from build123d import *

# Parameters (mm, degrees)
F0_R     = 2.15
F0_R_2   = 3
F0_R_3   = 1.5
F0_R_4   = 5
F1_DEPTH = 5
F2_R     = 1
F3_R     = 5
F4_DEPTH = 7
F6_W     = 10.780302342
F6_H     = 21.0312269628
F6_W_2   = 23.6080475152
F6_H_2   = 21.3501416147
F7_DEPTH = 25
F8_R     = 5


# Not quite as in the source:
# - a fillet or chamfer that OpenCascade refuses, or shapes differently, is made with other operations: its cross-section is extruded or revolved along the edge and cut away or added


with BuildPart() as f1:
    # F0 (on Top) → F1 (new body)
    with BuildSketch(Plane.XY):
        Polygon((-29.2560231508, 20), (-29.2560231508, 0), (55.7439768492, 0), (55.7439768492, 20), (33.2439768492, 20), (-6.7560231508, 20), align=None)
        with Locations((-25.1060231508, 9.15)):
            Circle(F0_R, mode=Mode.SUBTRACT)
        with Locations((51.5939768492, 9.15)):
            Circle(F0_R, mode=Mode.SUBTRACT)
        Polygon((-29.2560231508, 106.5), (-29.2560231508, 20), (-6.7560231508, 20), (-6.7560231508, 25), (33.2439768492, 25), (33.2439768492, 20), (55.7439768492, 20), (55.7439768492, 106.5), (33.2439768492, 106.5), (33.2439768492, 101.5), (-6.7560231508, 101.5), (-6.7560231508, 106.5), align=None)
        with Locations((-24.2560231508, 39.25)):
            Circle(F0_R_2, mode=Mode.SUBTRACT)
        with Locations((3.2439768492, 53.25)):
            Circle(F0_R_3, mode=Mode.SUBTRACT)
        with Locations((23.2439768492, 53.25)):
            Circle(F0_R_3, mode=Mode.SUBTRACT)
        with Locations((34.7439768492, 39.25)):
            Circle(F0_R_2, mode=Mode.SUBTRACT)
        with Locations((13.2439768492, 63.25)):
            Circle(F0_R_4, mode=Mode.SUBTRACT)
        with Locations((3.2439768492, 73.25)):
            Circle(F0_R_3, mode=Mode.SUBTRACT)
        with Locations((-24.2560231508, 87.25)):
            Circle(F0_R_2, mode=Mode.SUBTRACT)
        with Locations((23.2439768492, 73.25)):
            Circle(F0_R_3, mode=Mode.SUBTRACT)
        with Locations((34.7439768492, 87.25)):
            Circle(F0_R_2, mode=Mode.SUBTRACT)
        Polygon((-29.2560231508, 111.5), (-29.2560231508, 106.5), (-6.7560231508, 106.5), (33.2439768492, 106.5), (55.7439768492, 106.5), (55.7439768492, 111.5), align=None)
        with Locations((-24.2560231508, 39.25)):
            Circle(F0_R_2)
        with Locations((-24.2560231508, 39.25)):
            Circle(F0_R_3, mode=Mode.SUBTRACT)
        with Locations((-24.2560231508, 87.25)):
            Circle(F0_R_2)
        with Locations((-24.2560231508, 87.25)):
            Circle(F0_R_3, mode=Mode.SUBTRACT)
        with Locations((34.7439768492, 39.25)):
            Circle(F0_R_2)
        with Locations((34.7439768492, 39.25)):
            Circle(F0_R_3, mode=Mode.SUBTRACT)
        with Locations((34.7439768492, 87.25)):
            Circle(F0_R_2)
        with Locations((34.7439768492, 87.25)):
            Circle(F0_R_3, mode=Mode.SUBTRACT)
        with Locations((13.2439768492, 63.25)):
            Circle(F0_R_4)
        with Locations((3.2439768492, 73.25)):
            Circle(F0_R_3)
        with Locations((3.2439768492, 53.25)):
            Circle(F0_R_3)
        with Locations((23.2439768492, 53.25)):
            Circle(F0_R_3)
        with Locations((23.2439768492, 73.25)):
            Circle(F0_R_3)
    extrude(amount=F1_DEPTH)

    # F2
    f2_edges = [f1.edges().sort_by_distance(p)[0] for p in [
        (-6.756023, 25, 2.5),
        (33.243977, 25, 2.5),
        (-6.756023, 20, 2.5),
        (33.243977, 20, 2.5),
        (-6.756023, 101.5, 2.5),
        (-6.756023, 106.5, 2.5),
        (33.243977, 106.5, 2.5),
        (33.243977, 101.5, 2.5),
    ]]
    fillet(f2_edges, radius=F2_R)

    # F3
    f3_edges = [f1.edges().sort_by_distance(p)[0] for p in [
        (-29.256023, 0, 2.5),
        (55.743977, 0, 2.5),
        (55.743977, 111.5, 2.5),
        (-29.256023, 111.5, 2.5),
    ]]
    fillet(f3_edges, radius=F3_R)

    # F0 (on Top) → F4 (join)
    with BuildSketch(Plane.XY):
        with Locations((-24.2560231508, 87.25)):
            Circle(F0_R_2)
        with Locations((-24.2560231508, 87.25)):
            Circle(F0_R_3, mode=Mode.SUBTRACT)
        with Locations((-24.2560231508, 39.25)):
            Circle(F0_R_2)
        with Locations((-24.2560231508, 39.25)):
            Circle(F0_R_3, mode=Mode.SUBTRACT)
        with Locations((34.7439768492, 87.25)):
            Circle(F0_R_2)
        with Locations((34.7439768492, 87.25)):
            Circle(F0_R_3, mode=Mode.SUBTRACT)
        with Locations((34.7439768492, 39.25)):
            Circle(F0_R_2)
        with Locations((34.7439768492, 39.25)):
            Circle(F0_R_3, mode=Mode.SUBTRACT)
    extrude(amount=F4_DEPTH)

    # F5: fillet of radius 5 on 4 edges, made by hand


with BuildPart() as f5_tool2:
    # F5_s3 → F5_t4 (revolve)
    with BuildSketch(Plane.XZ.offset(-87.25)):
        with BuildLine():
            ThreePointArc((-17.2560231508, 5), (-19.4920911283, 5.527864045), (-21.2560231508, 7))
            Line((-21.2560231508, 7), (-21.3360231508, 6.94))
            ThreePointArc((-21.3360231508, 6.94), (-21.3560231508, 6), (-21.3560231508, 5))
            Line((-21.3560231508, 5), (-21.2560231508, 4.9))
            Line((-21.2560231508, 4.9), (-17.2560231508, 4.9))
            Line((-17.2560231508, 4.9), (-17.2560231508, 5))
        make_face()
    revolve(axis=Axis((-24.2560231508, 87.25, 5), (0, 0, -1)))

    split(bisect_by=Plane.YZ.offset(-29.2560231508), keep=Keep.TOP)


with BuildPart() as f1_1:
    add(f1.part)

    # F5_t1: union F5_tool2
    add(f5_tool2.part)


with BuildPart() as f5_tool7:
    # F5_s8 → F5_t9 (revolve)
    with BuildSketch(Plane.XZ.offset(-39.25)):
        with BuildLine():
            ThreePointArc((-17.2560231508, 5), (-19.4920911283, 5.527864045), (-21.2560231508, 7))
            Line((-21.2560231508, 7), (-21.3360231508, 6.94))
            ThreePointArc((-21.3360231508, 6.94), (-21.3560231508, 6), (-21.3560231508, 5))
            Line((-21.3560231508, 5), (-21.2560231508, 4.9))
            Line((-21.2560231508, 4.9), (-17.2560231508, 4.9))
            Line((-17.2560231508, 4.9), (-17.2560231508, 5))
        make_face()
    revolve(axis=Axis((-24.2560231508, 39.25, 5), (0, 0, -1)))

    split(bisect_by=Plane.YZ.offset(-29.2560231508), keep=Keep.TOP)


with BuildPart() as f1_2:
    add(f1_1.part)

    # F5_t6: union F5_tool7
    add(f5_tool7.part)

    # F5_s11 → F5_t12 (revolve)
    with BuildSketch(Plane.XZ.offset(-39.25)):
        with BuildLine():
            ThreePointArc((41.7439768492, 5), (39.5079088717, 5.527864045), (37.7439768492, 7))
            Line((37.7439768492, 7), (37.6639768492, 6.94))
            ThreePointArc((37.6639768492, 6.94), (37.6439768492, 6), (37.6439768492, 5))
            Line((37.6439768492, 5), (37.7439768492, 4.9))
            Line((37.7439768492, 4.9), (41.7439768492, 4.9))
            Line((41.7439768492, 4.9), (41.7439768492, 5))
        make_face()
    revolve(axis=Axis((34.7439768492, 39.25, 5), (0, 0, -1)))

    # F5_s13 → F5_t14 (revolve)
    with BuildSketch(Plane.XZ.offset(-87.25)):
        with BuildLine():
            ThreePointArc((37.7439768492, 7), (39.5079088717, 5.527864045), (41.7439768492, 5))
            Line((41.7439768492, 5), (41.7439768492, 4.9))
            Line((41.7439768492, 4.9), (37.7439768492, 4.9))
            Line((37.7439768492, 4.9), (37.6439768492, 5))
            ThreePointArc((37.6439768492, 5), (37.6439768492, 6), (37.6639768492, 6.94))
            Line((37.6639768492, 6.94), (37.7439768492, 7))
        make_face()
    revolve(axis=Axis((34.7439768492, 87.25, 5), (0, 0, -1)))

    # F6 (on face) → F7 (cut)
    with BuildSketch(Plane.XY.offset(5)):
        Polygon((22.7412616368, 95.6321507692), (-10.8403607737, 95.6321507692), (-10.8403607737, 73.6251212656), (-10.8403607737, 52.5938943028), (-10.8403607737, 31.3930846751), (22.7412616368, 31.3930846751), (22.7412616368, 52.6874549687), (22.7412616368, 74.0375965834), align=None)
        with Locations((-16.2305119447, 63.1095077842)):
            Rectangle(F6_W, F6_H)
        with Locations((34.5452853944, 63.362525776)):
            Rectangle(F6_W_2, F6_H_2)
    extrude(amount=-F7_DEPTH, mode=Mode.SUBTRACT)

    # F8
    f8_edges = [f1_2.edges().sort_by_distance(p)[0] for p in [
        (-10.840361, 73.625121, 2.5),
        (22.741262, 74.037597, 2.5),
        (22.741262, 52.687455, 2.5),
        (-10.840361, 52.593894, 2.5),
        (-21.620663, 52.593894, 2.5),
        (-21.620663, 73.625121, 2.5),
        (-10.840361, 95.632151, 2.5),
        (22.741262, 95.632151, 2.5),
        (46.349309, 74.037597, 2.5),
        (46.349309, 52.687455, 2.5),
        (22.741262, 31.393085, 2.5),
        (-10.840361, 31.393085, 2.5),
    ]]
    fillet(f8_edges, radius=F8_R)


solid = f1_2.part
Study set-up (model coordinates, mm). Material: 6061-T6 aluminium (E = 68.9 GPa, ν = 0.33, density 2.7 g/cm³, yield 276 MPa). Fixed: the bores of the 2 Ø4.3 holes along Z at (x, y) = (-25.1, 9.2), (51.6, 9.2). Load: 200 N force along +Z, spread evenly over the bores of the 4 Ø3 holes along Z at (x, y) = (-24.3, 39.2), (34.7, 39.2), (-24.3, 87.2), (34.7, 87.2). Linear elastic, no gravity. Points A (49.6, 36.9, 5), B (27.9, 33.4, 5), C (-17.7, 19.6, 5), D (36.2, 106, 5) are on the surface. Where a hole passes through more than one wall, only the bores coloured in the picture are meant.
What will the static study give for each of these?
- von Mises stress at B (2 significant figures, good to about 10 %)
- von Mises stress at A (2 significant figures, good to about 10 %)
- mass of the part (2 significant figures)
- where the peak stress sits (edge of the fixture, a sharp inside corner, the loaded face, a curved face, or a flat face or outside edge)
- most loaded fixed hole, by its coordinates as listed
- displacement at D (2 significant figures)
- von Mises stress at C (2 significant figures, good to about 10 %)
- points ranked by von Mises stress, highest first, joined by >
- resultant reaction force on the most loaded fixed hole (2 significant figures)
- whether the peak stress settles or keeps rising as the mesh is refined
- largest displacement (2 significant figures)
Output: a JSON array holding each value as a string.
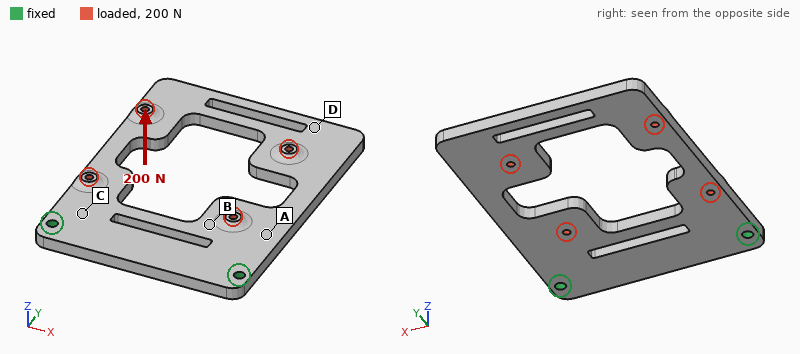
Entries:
["13 MPa", "26 MPa", "84 g", "edge of the fixture", "(-25.1, 9.2)", "0.96 mm", "44 MPa", "C > A > B > D", "120 N", "keeps rising", "1.1 mm"]
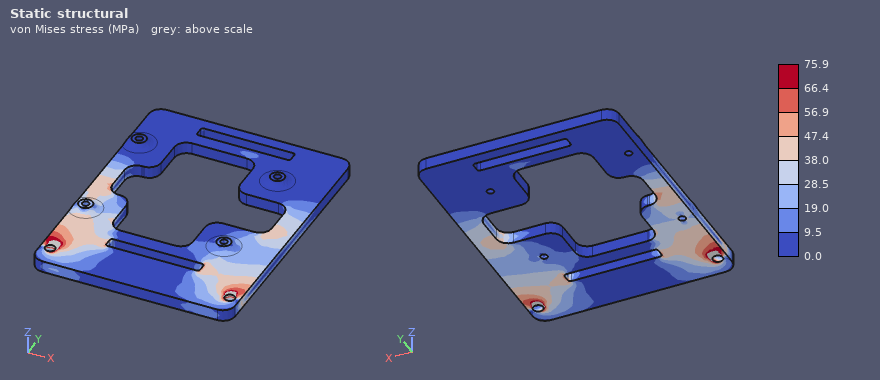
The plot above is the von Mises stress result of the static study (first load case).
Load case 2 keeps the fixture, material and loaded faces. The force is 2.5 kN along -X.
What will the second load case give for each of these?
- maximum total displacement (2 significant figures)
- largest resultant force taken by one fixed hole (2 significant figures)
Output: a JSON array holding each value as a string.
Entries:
["0.37 mm", "2.1 kN"]
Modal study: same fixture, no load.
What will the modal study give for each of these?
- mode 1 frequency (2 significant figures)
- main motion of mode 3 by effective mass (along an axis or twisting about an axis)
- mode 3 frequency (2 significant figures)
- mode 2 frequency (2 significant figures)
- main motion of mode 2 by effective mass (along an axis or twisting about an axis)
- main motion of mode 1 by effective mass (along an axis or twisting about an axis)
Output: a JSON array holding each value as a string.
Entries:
["300 Hz", "along X", "1800 Hz", "800 Hz", "twisting about Y", "along Z"]
